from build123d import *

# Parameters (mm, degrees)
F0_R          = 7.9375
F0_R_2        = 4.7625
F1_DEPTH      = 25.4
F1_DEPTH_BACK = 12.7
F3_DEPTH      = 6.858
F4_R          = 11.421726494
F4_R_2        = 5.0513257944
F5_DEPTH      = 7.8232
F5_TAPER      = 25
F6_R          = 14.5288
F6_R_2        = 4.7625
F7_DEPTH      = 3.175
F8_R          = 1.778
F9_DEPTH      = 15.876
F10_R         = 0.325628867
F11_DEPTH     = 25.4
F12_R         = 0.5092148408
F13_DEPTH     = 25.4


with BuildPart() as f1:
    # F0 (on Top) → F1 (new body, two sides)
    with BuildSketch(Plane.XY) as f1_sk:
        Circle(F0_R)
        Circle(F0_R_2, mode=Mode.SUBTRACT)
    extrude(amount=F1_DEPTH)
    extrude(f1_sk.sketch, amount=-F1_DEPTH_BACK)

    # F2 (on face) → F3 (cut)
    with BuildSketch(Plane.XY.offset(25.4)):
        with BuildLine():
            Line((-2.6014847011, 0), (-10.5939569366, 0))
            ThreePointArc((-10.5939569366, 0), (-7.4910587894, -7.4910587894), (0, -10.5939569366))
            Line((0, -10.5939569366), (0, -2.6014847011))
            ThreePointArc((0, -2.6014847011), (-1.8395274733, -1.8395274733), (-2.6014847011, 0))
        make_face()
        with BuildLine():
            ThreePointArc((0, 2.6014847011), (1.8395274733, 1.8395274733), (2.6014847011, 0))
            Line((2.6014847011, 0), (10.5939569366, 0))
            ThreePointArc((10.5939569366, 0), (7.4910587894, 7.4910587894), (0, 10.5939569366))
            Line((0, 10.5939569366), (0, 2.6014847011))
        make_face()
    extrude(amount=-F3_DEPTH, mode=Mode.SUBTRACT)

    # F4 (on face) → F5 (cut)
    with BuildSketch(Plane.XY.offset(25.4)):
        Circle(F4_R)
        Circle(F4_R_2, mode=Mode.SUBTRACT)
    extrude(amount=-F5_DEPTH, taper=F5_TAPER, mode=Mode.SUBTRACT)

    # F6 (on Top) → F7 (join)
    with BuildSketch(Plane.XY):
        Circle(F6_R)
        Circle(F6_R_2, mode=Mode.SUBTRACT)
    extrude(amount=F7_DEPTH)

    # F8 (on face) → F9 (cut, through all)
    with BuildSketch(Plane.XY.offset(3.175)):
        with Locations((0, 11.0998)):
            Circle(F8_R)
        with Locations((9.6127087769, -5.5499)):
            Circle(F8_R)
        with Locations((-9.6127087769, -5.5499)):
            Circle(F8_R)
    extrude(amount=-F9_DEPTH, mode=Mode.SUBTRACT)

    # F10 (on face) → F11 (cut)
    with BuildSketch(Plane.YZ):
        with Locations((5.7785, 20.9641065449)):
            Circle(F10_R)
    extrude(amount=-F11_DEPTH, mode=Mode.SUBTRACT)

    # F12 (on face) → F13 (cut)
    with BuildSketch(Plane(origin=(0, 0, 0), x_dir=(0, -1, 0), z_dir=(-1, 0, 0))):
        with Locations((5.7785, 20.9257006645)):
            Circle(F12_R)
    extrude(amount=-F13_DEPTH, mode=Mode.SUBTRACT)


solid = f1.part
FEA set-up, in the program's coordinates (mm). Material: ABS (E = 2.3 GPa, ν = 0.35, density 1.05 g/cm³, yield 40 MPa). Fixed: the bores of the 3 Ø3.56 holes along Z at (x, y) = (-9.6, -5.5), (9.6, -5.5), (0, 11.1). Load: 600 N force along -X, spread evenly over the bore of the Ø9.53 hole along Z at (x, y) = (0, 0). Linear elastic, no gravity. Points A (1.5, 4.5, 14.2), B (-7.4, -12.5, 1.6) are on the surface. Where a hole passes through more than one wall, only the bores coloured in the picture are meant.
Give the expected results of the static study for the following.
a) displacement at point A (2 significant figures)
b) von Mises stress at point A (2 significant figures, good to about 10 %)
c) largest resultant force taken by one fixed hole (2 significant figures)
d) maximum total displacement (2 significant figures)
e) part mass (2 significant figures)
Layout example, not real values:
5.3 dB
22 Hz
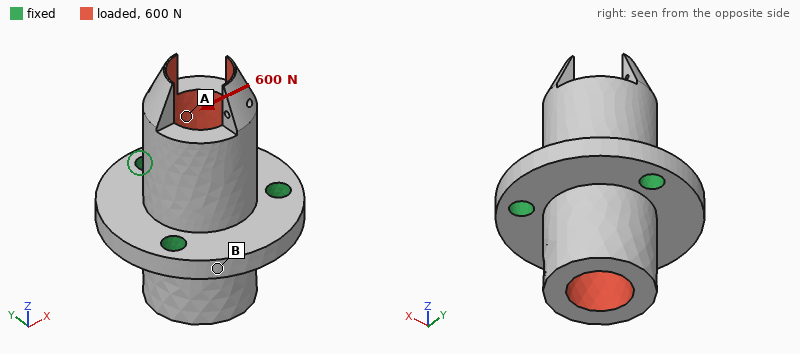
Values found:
0.12 mm
5.1 MPa
230 N
0.29 mm
5.9 g
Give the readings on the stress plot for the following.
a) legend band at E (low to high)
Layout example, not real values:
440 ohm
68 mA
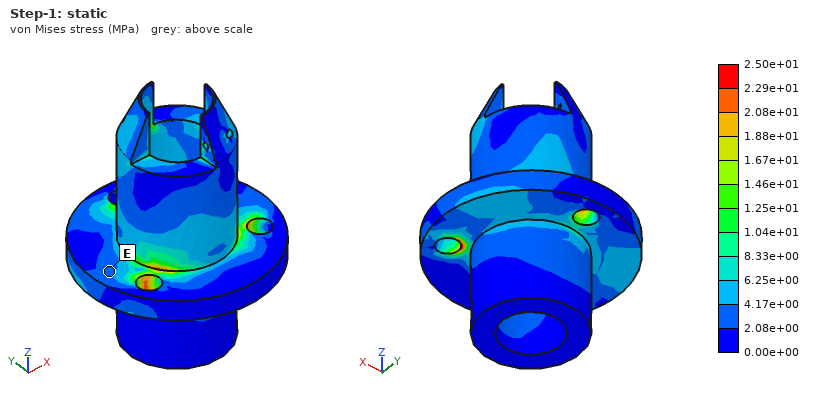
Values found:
2.08e+00 to 4.17e+00 MPa
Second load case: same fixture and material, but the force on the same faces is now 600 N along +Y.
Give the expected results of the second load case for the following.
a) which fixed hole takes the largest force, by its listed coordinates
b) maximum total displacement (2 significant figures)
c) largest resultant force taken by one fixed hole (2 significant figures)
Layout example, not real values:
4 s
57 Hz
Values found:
(0, 11.1)
0.29 mm
240 N
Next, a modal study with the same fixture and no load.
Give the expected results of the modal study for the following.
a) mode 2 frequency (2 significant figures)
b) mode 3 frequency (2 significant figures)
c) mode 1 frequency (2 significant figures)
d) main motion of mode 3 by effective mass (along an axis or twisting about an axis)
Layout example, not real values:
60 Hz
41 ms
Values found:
4600 Hz
8100 Hz
4500 Hz
along Z
